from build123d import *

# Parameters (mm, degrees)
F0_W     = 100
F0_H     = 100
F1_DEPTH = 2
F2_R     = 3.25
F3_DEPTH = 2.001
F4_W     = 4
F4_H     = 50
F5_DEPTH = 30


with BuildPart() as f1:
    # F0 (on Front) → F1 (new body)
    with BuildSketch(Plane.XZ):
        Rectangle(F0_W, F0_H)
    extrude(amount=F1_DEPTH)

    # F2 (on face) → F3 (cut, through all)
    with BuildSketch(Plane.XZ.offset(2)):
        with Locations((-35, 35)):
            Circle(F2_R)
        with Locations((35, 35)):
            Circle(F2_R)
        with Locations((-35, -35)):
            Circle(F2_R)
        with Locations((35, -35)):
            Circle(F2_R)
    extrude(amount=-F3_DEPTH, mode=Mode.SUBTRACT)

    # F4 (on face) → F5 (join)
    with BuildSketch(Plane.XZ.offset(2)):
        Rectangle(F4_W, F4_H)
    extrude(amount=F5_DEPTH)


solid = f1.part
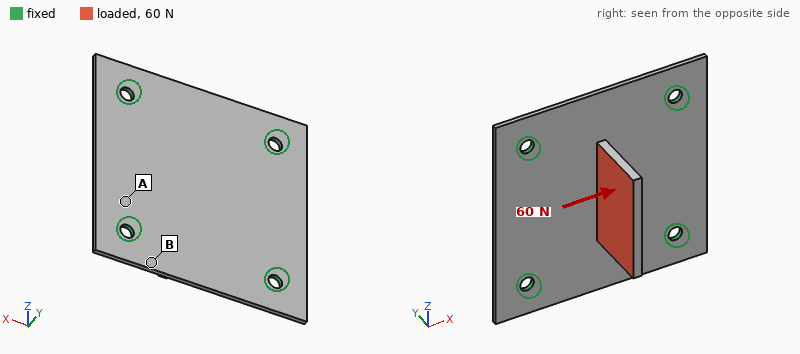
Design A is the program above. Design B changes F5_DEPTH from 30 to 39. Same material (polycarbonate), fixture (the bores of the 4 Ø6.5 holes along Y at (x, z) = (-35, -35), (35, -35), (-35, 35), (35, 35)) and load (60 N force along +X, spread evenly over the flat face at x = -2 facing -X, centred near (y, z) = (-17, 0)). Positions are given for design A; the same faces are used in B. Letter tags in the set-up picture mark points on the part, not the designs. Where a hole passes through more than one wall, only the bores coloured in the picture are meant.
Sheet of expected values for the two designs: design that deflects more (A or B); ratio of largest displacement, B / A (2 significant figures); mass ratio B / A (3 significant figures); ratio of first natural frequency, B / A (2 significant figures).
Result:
B
1.8
1.07
0.82
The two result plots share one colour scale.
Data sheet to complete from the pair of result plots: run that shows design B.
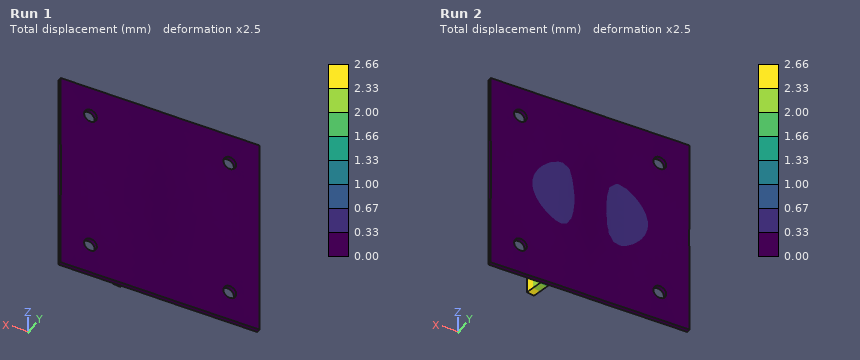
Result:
Run 2
